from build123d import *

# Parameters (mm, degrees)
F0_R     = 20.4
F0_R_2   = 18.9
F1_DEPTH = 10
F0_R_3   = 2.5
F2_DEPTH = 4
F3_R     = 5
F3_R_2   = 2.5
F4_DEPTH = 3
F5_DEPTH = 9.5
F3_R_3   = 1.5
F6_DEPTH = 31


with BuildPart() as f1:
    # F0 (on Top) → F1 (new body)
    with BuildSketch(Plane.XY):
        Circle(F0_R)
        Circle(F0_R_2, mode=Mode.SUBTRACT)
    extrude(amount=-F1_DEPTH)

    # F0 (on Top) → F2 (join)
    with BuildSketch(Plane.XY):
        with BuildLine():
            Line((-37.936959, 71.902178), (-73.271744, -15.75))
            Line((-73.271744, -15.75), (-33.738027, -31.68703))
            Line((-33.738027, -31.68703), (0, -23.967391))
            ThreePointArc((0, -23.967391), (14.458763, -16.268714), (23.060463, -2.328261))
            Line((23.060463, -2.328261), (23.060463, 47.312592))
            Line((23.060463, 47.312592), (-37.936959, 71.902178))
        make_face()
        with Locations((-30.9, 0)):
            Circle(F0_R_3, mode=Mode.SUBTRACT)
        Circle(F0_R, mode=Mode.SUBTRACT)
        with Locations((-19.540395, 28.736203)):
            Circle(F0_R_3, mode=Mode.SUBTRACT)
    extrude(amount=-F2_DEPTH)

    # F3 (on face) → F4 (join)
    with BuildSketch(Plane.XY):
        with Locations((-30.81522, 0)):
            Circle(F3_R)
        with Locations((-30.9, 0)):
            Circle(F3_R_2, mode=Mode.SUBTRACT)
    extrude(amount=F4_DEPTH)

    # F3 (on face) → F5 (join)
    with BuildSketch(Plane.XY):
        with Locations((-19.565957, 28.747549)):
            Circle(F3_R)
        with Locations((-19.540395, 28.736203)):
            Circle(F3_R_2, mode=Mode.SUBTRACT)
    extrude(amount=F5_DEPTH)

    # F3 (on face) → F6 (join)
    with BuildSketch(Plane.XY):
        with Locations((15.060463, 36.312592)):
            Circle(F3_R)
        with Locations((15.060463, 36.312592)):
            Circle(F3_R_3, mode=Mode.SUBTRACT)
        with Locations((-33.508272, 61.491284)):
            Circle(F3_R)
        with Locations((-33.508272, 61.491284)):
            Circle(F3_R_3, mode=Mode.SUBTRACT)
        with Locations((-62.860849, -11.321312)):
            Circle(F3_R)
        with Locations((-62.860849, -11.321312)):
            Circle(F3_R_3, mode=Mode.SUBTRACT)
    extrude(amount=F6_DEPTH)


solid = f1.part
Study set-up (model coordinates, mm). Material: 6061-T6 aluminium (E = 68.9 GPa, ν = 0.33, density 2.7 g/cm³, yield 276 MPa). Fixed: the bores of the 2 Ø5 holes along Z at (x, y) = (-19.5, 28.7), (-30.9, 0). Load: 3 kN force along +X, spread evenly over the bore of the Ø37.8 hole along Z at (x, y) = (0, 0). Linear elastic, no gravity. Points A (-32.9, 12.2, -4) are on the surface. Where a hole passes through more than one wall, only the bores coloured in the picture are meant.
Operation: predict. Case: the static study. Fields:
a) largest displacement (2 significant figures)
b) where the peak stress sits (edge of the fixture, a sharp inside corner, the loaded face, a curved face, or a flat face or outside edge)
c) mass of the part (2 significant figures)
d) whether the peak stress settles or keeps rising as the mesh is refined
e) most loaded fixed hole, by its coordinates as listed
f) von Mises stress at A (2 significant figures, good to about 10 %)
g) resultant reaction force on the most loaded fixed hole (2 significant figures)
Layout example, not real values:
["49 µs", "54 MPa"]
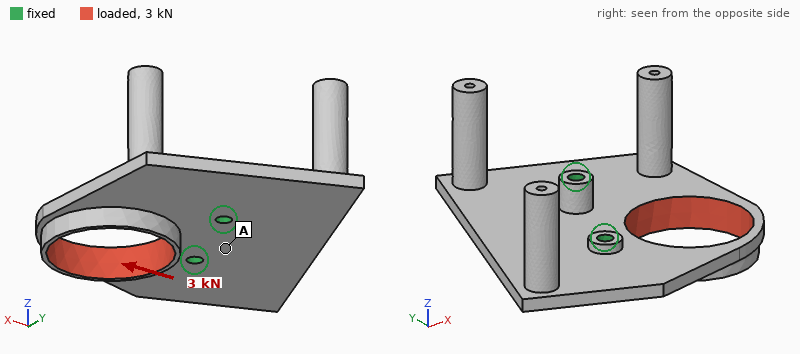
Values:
["0.35 mm", "edge of the fixture", "85 g", "keeps rising", "(-30.9, 0)", "12 MPa", "2.8 kN"]
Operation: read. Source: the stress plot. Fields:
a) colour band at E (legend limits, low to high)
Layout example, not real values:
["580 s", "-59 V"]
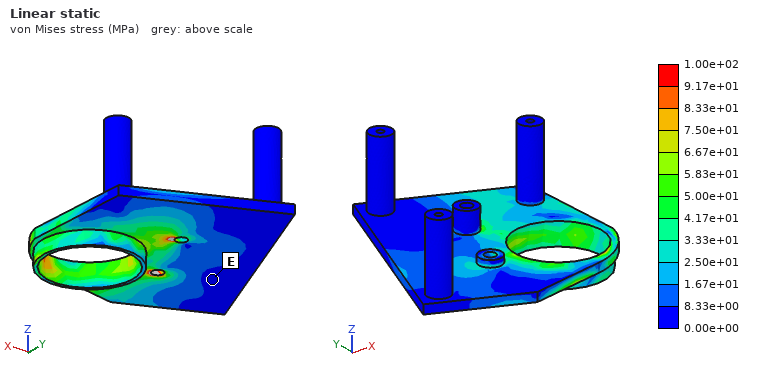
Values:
["0.00e+00 to 8.33e+00 MPa"]
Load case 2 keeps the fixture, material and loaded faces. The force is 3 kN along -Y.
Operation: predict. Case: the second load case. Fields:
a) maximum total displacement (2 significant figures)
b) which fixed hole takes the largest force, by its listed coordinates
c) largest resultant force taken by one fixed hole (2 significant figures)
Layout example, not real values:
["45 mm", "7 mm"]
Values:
["0.23 mm", "(-19.5, 28.7)", "3.0 kN"]
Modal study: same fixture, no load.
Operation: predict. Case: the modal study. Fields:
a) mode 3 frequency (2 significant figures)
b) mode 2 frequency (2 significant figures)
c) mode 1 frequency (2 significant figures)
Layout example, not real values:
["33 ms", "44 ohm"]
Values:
["1500 Hz", "1500 Hz", "1300 Hz"]
